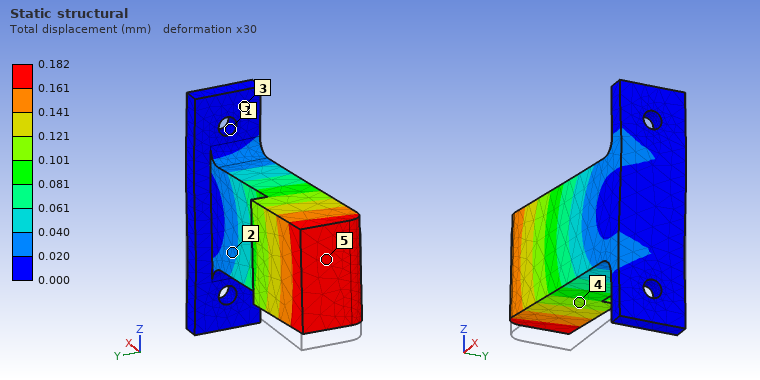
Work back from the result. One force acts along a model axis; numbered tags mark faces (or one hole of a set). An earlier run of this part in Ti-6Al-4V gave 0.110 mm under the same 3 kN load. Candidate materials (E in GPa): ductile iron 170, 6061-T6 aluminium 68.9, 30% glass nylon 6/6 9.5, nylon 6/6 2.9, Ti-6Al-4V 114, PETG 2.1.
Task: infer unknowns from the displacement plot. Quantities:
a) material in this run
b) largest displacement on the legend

6061-T6 aluminium
0.182 mm
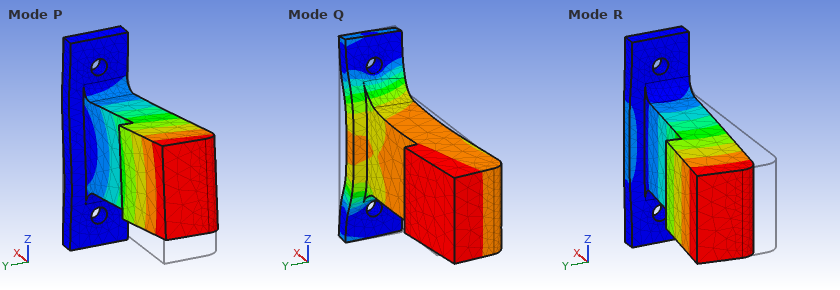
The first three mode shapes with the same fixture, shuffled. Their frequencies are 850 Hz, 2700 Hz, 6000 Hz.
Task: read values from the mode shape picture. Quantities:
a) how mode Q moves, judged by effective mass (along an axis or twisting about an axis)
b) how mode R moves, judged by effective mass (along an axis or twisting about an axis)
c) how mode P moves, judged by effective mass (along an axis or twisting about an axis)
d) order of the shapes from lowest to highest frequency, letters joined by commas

along X
along Y
along Z
R, P, Q
